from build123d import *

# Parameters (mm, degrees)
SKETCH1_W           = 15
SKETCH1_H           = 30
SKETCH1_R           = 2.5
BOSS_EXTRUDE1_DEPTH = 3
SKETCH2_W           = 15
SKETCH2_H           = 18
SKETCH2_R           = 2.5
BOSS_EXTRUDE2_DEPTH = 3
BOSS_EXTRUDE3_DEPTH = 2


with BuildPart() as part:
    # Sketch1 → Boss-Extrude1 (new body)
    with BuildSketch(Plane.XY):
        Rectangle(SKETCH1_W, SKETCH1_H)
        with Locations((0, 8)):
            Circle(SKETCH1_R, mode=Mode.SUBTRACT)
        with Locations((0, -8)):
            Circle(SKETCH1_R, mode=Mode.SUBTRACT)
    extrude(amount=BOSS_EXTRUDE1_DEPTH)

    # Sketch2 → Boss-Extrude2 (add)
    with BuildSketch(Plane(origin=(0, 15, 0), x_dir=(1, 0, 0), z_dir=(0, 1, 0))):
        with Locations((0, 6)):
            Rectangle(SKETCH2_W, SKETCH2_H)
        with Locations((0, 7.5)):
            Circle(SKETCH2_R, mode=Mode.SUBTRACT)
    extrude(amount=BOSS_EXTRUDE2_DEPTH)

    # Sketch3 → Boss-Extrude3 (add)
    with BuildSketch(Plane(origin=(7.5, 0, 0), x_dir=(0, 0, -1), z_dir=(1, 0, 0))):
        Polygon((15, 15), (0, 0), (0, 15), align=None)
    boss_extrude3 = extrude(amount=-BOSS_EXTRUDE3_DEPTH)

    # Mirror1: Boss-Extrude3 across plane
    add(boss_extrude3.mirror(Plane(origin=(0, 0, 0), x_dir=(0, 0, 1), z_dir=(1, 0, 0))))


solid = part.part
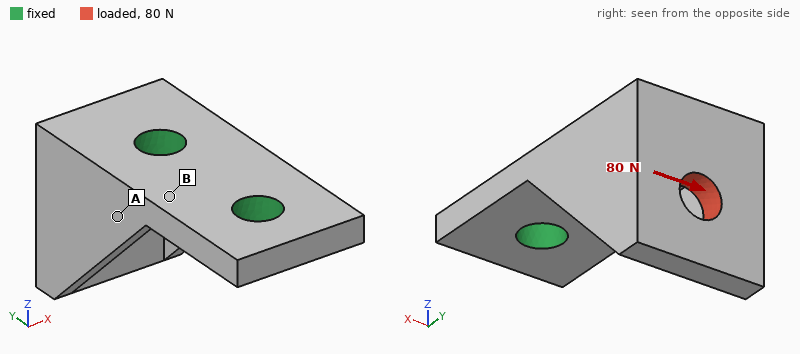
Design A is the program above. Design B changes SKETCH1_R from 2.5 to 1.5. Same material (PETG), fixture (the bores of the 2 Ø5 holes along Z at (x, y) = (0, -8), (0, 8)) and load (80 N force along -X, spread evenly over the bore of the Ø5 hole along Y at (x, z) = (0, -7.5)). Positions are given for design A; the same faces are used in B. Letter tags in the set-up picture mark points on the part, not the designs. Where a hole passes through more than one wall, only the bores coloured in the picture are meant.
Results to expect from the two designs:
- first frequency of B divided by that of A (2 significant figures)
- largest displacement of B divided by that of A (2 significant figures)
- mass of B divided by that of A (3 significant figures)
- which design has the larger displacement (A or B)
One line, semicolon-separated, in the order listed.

0.83; 1.4; 1.03; B
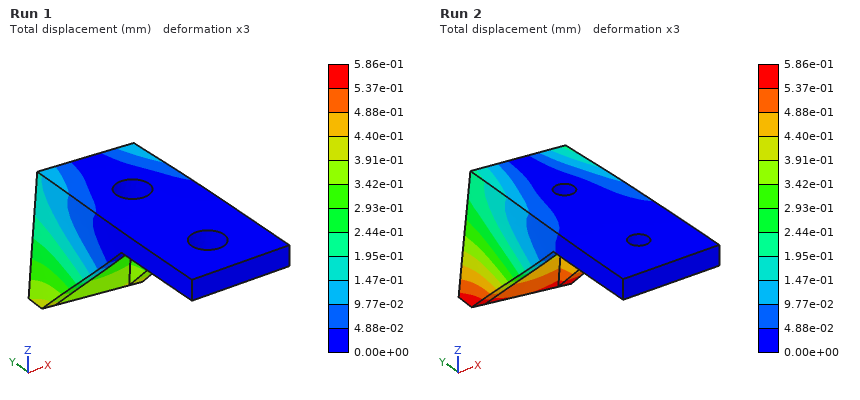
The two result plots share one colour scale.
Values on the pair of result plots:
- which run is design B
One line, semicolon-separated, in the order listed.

Run 2
